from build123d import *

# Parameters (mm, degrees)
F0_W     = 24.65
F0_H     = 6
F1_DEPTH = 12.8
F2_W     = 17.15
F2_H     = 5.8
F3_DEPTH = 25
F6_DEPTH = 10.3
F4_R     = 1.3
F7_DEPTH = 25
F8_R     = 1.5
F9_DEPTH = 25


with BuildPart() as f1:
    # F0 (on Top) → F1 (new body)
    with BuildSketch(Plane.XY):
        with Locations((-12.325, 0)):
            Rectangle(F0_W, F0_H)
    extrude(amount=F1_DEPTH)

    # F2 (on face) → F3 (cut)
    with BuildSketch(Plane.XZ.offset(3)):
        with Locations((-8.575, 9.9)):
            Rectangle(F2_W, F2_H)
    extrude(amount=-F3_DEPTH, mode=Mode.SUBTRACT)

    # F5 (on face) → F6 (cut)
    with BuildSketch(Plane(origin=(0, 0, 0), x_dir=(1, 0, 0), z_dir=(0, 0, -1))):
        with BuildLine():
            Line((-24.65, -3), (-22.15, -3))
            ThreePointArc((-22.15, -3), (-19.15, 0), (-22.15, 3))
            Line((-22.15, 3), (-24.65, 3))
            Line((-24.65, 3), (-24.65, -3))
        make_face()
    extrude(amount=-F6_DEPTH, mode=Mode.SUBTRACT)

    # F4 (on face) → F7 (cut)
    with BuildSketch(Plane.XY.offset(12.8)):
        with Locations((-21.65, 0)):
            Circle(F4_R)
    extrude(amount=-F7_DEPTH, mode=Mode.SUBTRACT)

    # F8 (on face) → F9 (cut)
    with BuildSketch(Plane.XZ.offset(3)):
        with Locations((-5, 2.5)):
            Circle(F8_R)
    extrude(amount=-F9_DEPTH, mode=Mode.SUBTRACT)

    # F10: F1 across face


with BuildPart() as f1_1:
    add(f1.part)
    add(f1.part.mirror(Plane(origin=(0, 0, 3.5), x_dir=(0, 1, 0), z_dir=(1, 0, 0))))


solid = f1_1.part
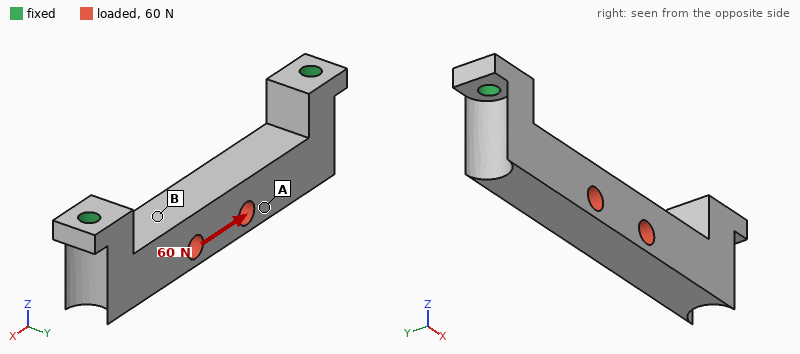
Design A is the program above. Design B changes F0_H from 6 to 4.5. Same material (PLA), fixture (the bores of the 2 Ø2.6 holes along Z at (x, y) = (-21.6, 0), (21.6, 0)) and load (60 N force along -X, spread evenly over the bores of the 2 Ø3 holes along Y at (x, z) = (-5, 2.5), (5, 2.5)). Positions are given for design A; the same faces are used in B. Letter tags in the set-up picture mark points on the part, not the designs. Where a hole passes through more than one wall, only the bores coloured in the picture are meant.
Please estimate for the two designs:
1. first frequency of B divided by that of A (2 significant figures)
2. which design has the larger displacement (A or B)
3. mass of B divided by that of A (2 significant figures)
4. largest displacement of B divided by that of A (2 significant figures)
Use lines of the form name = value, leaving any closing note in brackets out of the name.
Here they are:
first frequency of B divided by that of A = 0.79
which design has the larger displacement = B
mass of B divided by that of A = 0.73
largest displacement of B divided by that of A = 1.6
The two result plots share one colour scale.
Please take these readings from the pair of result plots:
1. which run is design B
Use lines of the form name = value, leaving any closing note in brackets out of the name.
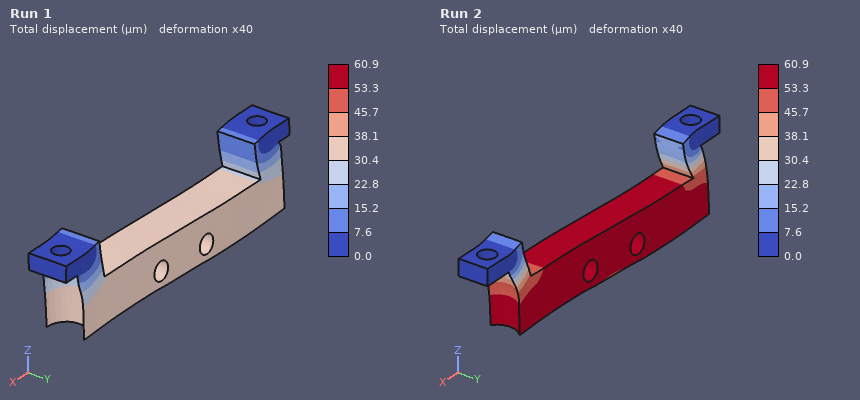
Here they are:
which run is design B = Run 2
